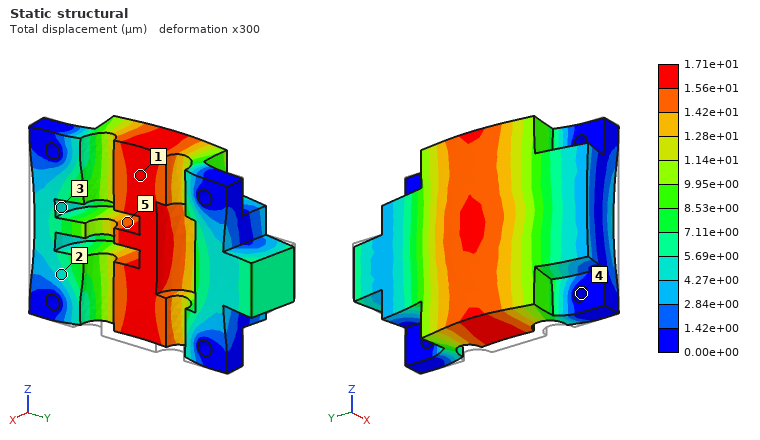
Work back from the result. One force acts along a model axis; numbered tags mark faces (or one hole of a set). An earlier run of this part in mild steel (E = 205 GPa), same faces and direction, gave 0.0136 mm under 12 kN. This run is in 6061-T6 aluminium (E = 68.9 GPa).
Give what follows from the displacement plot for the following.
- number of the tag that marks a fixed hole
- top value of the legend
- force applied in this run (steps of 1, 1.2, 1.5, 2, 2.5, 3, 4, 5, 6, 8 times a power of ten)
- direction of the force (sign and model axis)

4
1.71e+01 µm
5 kN
-X
